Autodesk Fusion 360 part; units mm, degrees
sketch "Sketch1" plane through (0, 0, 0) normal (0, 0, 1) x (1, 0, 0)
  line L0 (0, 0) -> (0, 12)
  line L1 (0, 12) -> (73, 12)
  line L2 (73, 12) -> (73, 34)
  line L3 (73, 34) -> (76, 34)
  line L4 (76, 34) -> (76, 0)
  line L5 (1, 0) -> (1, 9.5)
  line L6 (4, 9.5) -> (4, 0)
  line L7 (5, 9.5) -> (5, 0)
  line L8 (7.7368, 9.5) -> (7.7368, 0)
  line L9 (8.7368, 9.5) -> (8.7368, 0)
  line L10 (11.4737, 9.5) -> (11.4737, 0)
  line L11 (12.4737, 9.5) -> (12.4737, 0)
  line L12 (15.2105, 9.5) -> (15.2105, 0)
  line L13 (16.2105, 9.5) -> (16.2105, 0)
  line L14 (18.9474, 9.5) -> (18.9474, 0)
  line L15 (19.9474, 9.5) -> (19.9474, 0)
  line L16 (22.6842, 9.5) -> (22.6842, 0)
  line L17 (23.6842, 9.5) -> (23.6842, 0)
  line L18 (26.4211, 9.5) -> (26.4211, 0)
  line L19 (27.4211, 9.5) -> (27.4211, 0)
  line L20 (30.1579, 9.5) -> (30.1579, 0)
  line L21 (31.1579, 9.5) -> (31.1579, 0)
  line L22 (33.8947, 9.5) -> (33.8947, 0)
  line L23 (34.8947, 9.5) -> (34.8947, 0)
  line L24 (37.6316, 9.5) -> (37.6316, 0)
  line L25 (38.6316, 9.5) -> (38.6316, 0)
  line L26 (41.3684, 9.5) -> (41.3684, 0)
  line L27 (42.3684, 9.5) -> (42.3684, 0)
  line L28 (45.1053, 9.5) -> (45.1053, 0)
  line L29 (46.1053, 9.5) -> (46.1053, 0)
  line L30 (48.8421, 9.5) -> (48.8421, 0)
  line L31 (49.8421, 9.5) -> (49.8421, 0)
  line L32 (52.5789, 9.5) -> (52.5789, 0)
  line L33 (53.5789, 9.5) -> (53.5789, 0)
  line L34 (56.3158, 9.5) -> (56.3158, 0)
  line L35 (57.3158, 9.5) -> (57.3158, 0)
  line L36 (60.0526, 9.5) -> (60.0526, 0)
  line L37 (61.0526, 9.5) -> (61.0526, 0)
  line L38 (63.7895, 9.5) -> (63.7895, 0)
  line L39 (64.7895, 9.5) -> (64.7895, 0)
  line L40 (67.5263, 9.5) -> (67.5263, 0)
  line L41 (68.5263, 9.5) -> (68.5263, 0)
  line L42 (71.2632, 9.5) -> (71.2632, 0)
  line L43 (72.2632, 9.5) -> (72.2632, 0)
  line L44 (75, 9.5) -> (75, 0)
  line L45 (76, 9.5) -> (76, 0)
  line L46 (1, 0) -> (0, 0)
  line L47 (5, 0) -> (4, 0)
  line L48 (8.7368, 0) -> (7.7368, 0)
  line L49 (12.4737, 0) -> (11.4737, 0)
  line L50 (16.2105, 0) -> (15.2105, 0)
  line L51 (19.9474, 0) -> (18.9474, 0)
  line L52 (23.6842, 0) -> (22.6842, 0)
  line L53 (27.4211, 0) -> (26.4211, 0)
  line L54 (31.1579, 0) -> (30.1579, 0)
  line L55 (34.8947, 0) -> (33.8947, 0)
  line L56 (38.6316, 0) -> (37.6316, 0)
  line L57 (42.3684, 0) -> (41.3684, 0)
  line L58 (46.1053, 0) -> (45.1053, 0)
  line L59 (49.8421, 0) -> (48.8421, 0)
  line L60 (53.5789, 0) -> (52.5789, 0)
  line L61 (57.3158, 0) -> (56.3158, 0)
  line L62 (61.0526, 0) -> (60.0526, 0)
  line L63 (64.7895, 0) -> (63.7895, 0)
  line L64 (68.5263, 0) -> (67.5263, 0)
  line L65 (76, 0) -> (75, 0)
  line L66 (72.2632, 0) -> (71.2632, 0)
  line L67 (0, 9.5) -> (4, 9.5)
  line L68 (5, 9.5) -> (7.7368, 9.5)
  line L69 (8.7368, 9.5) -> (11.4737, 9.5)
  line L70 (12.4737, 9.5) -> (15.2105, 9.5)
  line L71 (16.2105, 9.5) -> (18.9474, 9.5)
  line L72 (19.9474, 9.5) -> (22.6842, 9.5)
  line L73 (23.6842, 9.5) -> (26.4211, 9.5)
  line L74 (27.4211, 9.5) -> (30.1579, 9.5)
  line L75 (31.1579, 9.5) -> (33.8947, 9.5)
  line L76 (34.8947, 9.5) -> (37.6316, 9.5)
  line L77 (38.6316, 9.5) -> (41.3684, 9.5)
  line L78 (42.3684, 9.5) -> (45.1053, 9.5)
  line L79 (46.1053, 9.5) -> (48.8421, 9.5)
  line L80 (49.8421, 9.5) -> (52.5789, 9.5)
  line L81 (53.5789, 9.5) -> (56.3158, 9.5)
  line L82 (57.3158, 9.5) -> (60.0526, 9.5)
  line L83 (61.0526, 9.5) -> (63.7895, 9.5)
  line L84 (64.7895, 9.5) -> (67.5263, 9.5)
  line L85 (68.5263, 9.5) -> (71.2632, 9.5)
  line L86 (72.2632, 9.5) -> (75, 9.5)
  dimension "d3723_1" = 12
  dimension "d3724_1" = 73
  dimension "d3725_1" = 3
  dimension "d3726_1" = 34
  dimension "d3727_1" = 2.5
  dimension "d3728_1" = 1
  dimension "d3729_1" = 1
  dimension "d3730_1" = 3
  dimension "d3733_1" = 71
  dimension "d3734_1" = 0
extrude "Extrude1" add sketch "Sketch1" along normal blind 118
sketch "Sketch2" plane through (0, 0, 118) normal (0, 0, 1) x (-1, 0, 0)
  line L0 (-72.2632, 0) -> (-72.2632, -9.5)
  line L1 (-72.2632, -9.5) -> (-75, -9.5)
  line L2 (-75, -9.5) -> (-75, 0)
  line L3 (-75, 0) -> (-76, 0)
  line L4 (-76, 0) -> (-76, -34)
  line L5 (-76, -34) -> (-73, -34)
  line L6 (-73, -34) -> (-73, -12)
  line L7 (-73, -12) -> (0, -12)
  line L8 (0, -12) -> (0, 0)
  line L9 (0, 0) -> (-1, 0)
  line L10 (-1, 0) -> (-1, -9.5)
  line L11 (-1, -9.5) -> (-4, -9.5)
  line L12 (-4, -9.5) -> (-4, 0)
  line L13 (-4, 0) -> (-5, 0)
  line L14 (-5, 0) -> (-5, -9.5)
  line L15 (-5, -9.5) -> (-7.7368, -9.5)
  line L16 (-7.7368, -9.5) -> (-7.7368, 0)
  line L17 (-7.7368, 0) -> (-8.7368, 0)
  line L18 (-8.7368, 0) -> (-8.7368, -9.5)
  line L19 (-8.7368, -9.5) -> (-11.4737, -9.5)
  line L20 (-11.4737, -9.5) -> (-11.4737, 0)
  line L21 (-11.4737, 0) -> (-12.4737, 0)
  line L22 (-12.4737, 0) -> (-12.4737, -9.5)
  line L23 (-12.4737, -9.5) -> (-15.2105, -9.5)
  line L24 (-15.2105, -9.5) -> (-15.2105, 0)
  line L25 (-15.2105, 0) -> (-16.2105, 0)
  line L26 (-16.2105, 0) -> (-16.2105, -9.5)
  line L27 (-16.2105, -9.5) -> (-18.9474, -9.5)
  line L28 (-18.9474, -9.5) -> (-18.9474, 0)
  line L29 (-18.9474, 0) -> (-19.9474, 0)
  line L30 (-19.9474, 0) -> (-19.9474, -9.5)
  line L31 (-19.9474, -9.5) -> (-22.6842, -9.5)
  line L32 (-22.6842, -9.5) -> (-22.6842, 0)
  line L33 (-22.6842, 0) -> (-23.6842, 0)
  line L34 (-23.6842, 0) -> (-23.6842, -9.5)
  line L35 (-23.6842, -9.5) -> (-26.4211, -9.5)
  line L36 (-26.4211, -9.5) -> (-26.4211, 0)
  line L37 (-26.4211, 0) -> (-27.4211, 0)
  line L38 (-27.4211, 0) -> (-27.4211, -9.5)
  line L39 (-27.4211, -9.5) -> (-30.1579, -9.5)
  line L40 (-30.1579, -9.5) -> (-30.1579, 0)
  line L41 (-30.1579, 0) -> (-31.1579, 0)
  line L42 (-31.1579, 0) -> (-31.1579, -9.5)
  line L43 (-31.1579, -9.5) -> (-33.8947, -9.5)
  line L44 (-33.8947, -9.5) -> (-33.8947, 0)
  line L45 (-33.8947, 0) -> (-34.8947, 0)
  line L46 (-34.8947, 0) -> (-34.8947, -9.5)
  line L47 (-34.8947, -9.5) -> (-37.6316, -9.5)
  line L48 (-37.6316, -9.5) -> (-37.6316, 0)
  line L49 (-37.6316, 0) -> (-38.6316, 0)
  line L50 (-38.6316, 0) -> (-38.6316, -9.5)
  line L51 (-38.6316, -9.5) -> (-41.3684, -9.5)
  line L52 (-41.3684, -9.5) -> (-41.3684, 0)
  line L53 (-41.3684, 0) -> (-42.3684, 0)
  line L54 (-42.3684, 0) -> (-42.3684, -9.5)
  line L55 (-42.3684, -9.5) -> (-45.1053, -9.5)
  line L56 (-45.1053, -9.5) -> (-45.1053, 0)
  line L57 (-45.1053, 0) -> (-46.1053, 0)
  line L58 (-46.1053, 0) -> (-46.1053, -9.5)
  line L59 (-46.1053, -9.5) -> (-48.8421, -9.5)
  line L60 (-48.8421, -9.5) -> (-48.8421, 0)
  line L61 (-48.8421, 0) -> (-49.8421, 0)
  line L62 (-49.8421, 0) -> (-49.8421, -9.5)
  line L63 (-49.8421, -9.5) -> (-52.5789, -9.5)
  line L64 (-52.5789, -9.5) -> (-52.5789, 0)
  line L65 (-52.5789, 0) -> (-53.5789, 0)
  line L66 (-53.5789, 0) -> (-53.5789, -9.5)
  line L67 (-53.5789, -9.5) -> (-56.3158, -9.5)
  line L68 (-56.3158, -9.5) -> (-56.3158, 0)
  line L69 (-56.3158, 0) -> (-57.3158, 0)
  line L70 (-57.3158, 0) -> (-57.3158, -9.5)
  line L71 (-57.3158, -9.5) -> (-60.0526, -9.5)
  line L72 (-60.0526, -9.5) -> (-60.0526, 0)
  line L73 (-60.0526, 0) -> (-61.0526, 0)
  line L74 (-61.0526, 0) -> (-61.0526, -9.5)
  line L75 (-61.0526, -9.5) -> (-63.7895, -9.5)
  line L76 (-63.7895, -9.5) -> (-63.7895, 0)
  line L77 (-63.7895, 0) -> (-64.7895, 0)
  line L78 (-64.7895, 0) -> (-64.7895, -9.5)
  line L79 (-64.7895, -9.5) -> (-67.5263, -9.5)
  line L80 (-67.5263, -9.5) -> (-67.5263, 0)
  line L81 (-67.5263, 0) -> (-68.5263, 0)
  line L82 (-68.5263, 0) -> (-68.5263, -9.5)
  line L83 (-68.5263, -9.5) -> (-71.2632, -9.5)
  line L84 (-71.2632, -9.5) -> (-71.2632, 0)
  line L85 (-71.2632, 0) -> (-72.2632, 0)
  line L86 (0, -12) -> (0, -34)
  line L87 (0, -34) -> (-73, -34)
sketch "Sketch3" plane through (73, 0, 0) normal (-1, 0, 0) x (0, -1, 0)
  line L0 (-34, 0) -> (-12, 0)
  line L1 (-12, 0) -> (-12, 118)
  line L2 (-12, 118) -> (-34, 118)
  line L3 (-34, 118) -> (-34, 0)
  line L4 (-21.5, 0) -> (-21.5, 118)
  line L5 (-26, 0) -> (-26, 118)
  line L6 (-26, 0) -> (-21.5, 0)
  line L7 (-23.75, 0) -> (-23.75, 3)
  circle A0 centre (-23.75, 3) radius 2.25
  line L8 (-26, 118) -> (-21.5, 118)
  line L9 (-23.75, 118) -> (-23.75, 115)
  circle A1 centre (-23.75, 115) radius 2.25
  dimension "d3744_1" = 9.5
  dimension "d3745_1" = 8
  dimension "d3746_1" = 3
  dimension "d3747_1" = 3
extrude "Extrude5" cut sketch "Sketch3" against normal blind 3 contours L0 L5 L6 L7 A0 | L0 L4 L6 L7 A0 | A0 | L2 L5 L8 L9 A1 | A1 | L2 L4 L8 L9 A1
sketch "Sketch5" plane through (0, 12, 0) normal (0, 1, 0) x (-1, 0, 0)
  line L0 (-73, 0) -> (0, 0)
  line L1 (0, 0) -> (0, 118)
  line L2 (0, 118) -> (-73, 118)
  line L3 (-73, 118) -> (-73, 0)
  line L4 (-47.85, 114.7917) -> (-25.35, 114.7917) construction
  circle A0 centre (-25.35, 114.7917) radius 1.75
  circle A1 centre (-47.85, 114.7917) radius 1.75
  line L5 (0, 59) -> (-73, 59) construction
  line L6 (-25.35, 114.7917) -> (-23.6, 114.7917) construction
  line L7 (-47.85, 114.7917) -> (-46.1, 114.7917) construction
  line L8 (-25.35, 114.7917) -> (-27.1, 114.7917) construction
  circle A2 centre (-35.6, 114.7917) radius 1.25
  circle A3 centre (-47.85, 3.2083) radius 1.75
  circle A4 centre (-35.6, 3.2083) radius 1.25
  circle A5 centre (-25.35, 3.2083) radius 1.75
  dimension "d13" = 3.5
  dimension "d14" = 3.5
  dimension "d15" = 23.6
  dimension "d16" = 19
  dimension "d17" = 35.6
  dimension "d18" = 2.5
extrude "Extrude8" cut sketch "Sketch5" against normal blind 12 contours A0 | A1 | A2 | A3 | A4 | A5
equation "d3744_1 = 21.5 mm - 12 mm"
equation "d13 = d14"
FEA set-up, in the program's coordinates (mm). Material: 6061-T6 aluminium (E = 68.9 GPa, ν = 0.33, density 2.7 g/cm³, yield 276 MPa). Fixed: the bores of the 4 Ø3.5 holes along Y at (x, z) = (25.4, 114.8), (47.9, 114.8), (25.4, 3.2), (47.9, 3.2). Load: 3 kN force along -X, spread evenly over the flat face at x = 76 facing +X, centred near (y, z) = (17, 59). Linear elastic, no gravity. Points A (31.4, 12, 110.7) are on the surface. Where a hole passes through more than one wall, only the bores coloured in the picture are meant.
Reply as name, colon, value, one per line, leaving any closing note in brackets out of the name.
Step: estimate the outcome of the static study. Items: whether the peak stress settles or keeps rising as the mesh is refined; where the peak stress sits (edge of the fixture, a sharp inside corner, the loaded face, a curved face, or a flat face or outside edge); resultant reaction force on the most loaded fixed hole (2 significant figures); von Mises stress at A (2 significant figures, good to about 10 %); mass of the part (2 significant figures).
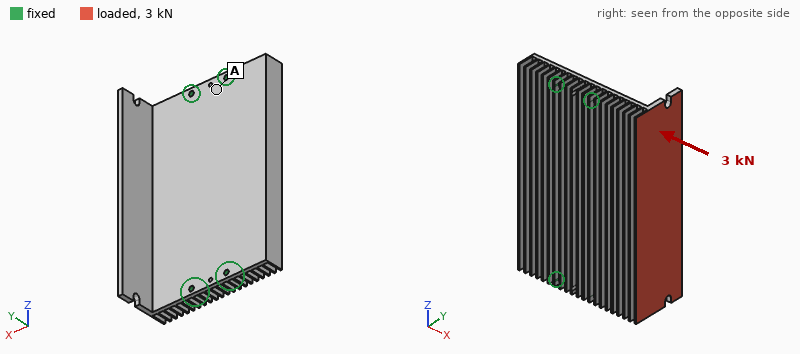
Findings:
whether the peak stress settles or keeps rising as the mesh is refined: keeps rising
where the peak stress sits: edge of the fixture
resultant reaction force on the most loaded fixed hole: 1000 N
von Mises stress at A: 16 MPa
mass of the part: 140 g
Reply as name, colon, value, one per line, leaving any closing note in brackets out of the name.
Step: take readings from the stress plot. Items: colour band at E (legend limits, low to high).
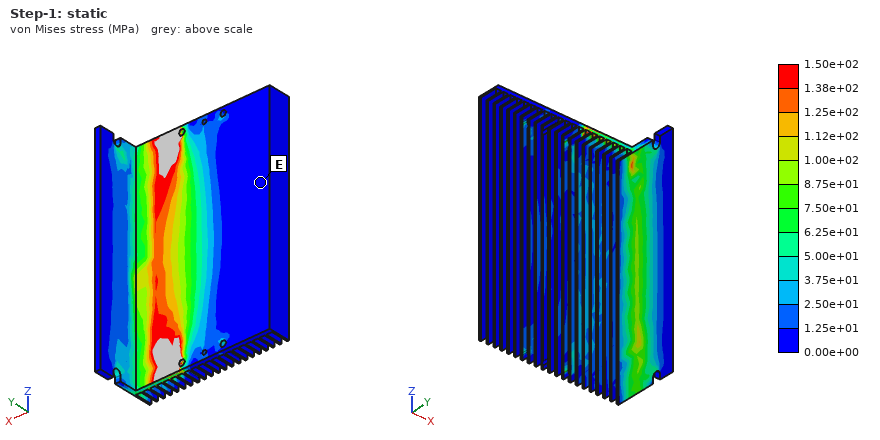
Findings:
colour band at E: 0.00e+00 to 1.25e+01 MPa
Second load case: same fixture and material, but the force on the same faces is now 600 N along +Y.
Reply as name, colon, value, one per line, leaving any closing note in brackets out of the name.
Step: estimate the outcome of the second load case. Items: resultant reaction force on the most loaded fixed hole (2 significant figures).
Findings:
resultant reaction force on the most loaded fixed hole: 490 N
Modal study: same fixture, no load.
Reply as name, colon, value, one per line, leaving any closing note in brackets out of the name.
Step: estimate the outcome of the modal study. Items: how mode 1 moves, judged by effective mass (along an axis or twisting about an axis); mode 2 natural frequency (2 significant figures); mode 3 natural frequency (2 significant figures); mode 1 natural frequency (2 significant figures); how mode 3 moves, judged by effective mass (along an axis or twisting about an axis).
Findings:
how mode 1 moves, judged by effective mass: along Y
mode 2 natural frequency: 1400 Hz
mode 3 natural frequency: 1600 Hz
mode 1 natural frequency: 820 Hz
how mode 3 moves, judged by effective mass: along Y
